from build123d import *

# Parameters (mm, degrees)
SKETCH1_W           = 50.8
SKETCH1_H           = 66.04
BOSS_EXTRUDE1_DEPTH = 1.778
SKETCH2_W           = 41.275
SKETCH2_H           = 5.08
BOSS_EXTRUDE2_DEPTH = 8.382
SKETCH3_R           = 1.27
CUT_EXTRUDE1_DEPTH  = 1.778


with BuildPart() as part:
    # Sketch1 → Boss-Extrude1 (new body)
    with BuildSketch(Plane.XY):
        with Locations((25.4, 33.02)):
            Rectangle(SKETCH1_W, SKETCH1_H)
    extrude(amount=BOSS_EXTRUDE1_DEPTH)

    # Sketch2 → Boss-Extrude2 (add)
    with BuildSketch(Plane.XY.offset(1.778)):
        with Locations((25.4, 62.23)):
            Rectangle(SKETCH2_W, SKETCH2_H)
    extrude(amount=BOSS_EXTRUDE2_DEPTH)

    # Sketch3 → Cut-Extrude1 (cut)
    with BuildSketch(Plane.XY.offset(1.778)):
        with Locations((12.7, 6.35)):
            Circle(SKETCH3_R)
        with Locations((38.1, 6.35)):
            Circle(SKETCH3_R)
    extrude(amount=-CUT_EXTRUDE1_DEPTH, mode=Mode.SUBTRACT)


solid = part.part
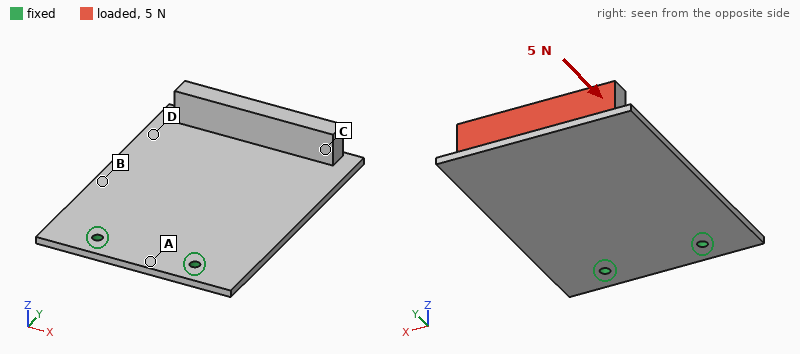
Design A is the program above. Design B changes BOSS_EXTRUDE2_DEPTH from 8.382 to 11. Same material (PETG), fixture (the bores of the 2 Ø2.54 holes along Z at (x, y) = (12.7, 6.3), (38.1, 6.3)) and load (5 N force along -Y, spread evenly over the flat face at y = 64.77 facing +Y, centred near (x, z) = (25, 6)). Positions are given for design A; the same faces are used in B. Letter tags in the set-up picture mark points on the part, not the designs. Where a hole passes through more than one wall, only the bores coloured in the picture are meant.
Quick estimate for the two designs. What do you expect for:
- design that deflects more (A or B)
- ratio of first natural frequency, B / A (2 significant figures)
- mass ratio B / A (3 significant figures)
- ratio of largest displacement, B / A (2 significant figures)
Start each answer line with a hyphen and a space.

- B
- 0.92
- 1.07
- 1.3
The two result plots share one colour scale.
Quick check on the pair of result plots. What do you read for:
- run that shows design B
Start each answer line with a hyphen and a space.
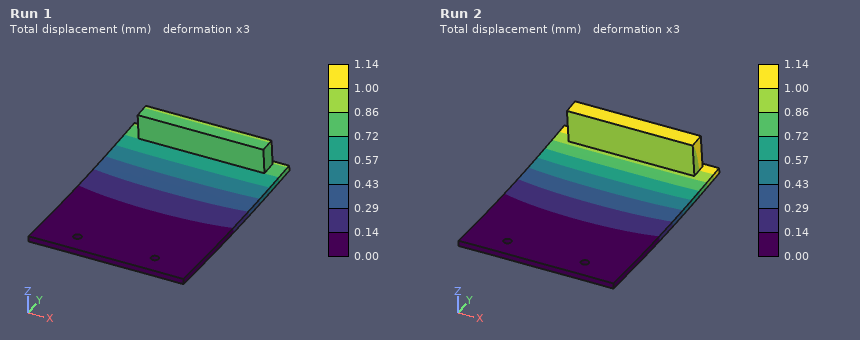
- Run 2
